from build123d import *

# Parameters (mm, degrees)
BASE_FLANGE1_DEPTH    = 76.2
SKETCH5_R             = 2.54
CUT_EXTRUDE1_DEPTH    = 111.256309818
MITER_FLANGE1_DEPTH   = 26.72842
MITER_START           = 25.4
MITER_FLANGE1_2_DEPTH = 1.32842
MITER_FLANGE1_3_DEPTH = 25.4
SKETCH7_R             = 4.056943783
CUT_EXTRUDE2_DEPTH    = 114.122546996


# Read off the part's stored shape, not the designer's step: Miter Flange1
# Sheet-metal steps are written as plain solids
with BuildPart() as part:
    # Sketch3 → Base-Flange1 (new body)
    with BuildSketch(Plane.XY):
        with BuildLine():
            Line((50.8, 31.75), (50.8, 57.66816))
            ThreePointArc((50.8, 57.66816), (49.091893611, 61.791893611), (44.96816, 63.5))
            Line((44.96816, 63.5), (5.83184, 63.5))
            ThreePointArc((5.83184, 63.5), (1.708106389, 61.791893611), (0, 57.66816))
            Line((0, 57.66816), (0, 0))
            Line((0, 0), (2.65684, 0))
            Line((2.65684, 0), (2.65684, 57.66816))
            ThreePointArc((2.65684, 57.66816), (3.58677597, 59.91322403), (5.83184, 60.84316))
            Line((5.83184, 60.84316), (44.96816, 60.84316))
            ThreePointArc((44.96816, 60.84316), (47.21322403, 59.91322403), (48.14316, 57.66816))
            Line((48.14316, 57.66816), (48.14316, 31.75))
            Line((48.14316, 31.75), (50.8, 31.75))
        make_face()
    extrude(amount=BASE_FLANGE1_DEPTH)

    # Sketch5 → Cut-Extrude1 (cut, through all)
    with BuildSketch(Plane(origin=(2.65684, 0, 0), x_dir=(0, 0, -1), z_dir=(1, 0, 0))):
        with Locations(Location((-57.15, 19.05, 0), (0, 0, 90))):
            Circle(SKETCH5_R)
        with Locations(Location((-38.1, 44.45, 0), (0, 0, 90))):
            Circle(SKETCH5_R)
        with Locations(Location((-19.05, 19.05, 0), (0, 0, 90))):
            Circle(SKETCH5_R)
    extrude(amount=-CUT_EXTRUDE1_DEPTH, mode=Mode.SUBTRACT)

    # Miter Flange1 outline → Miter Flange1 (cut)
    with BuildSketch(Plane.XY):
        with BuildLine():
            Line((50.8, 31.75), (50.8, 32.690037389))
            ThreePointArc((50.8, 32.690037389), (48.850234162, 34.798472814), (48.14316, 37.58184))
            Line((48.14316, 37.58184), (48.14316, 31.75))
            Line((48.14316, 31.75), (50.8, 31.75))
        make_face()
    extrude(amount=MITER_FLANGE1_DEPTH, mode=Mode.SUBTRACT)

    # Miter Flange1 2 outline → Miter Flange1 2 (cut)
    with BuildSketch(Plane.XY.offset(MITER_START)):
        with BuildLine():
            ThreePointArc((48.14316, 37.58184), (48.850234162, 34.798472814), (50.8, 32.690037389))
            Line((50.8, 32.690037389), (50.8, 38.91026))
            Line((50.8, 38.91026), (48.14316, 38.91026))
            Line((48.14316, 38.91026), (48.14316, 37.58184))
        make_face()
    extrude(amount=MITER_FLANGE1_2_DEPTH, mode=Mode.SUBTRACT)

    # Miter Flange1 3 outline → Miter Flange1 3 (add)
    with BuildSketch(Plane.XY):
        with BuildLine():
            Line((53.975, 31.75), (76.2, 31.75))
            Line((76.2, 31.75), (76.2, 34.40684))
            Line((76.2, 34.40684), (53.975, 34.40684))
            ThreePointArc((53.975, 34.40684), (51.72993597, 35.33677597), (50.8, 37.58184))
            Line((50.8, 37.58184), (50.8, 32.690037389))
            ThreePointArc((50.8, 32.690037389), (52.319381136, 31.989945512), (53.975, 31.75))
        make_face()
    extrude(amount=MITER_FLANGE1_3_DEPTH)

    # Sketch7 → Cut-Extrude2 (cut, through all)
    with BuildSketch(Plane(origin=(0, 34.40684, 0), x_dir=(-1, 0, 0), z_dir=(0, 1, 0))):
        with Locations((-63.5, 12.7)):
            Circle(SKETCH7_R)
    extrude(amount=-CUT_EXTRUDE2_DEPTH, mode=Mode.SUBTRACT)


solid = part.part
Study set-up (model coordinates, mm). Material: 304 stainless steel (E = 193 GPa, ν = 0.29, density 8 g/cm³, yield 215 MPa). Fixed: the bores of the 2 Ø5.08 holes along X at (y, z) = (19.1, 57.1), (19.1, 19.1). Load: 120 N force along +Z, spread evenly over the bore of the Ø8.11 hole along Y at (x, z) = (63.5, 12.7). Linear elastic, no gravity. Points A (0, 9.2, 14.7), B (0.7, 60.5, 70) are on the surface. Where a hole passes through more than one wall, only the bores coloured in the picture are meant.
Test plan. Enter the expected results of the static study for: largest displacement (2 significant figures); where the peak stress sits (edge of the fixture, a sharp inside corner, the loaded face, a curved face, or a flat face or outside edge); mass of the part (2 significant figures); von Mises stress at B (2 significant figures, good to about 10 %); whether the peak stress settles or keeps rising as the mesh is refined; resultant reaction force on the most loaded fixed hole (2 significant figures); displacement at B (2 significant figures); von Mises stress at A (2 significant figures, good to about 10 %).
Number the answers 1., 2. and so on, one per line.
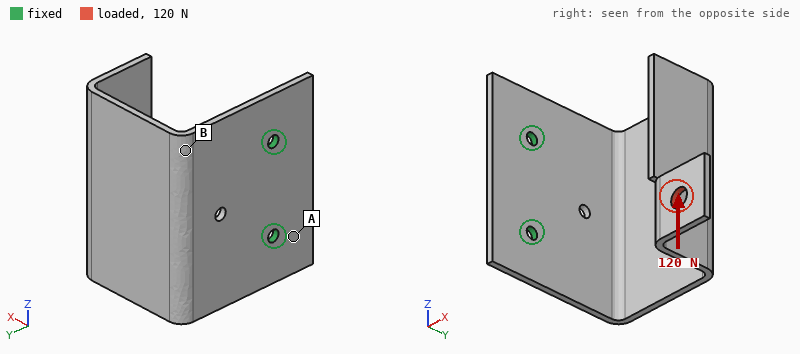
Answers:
1. 0.64 mm
2. edge of the fixture
3. 230 g
4. 43 MPa
5. keeps rising
6. 170 N
7. 0.16 mm
8. 8.5 MPa
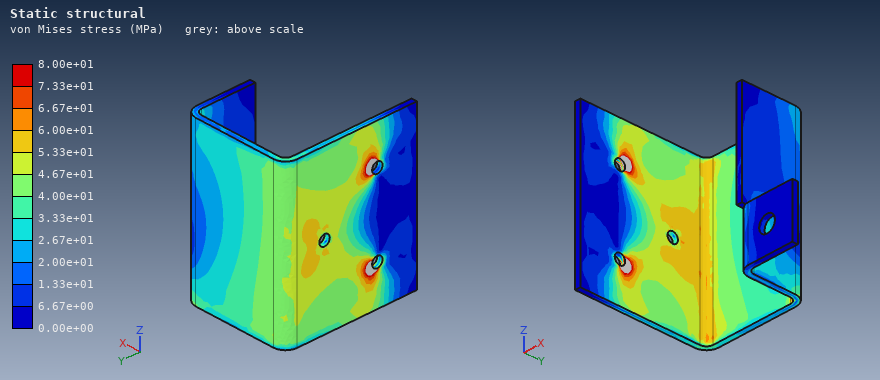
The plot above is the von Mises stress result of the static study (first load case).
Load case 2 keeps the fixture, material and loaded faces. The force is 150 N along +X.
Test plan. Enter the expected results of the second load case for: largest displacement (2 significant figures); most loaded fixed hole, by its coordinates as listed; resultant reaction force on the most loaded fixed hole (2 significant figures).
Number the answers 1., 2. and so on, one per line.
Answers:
1. 0.92 mm
2. (19.1, 19.1)
3. 150 N
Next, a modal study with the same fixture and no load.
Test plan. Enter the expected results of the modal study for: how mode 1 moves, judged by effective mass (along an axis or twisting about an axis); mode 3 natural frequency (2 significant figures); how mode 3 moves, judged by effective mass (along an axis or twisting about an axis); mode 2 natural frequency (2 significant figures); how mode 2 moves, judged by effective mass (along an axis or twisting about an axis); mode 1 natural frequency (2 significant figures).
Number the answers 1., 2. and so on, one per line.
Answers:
1. along Y
2. 490 Hz
3. along X
4. 330 Hz
5. along Z
6. 210 Hz
